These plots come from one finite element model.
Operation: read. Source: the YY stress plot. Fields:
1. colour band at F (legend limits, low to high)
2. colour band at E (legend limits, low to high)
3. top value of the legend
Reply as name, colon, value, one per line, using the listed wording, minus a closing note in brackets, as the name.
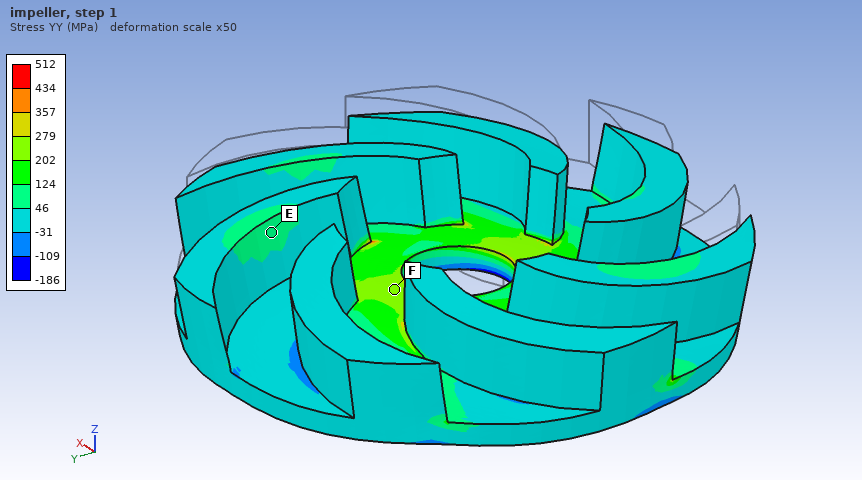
colour band at F: 202 to 279 MPa
colour band at E: 46 to 124 MPa
top value of the legend: 512 MPa
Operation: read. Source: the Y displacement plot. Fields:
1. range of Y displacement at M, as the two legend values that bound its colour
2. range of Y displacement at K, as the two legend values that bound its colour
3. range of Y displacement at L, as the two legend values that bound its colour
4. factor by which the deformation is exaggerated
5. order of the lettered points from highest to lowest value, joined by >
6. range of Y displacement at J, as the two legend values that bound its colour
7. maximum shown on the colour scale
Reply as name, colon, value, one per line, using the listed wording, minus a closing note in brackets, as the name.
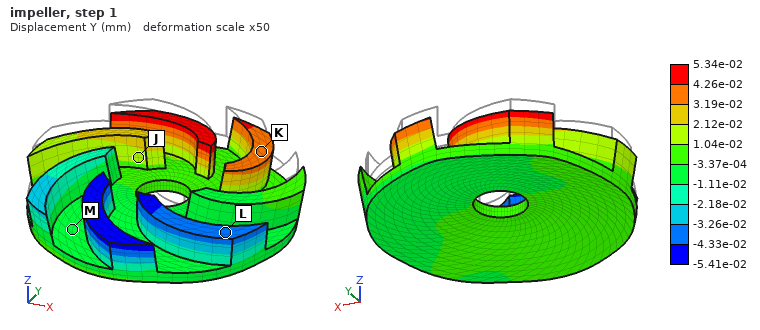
range of Y displacement at M, as the two legend values that bound its colour: -1.11e-02 to -3.37e-04 mm
range of Y displacement at K, as the two legend values that bound its colour: 3.19e-02 to 4.26e-02 mm
range of Y displacement at L, as the two legend values that bound its colour: -4.33e-02 to -3.26e-02 mm
factor by which the deformation is exaggerated: 50
order of the lettered points from highest to lowest value, joined by >: K > J > M > L
range of Y displacement at J, as the two legend values that bound its colour: 1.04e-02 to 2.12e-02 mm
maximum shown on the colour scale: 5.34e-02 mm
